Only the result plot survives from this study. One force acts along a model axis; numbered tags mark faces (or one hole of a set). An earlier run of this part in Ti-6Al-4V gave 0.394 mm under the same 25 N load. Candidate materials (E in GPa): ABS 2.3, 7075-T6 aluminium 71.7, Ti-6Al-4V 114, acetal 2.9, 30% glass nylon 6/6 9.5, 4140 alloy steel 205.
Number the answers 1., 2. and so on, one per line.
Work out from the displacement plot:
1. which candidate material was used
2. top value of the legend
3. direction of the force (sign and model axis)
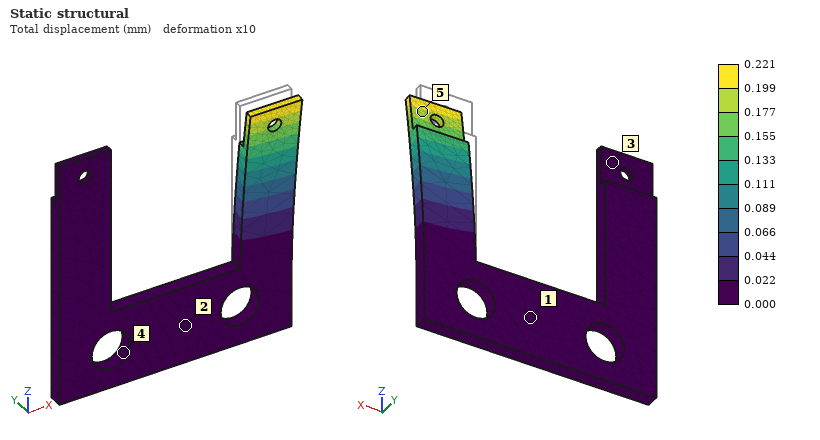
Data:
1. 4140 alloy steel
2. 0.221 mm
3. -Y
